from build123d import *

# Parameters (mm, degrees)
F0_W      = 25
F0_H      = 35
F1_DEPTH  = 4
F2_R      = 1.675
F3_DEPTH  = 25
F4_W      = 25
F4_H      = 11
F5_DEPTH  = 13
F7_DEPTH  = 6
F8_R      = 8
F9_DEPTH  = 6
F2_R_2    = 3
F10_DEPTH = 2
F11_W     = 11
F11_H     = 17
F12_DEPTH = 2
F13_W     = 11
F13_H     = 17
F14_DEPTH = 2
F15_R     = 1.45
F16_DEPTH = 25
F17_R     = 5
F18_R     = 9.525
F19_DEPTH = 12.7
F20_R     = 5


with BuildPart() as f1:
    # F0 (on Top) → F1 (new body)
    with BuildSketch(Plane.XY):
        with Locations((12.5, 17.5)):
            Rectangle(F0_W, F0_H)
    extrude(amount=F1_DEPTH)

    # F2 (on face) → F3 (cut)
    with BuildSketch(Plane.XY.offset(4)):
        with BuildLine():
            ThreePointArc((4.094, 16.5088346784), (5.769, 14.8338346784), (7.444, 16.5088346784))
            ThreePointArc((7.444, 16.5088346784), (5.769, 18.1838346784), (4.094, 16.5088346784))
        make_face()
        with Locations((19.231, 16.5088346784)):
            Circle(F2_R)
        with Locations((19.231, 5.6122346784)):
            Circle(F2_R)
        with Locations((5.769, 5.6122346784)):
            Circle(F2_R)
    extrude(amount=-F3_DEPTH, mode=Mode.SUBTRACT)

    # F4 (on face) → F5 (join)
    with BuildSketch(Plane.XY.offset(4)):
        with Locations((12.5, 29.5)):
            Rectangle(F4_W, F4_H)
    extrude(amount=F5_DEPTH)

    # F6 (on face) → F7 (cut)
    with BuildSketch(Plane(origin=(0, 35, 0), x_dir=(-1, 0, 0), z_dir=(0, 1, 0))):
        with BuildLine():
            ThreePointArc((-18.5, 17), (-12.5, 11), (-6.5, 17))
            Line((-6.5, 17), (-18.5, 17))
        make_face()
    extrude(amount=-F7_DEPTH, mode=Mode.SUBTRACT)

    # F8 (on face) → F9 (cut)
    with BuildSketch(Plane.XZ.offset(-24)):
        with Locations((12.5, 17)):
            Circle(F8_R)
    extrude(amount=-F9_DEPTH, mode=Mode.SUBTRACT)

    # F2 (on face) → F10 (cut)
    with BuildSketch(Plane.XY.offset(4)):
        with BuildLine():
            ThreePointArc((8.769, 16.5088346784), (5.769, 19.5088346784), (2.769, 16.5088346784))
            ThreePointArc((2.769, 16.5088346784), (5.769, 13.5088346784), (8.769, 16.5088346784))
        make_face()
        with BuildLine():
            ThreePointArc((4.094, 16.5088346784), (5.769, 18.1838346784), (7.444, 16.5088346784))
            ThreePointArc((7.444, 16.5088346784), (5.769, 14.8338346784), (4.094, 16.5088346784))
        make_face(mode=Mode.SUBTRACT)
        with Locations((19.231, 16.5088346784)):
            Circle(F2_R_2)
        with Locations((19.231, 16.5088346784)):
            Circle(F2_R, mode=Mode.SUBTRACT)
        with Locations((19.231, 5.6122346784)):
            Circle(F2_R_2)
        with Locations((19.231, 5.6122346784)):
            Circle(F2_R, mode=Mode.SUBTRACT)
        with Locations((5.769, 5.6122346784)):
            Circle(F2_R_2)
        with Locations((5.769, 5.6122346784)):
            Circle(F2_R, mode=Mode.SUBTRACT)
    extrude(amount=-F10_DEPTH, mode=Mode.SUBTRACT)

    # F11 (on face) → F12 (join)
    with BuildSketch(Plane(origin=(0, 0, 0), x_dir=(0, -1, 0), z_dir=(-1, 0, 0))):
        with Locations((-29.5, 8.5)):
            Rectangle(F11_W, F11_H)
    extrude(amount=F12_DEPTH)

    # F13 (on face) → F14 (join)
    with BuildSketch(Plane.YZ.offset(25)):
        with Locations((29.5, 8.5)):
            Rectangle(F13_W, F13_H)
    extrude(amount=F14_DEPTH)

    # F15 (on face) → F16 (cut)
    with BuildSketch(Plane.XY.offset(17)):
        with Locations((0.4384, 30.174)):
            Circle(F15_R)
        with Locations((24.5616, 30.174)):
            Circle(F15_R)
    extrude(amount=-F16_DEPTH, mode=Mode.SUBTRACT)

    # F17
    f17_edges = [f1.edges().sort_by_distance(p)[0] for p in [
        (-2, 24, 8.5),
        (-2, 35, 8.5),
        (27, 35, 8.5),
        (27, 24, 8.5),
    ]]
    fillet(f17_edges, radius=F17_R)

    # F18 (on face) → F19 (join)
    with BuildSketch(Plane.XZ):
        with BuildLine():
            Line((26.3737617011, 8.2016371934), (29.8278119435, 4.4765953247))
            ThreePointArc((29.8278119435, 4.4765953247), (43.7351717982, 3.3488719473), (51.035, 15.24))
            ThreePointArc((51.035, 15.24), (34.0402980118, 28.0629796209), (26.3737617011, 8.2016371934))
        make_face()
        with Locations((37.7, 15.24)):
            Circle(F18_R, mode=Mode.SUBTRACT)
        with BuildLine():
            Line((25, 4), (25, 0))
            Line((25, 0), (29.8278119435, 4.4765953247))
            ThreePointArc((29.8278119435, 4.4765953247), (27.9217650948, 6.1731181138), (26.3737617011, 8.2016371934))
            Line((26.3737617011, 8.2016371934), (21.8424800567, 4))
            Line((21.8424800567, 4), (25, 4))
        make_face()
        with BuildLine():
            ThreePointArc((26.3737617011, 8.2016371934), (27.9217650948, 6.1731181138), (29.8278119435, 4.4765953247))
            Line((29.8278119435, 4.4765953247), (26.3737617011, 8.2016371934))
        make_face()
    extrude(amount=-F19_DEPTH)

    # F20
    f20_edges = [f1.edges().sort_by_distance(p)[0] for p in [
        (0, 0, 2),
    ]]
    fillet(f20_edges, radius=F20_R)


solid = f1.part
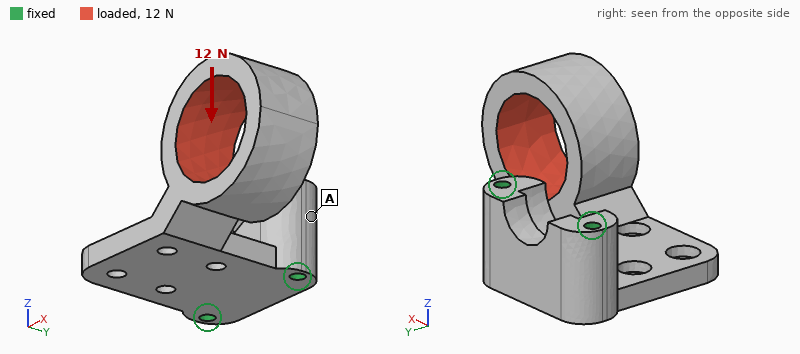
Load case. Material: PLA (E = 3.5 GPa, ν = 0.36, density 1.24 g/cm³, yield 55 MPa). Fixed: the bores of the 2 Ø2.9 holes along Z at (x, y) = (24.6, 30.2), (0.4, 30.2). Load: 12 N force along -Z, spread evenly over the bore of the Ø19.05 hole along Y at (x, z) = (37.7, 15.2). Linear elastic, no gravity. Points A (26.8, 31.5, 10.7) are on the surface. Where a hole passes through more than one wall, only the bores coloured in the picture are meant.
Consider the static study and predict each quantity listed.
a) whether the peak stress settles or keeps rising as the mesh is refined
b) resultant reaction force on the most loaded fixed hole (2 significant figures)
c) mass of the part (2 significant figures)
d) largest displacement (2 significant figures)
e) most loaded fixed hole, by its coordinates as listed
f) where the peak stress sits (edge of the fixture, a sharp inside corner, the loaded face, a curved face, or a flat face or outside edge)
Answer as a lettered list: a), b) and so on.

a) keeps rising
b) 21 N
c) 12 g
d) 0.67 mm
e) (24.6, 30.2)
f) a sharp inside corner
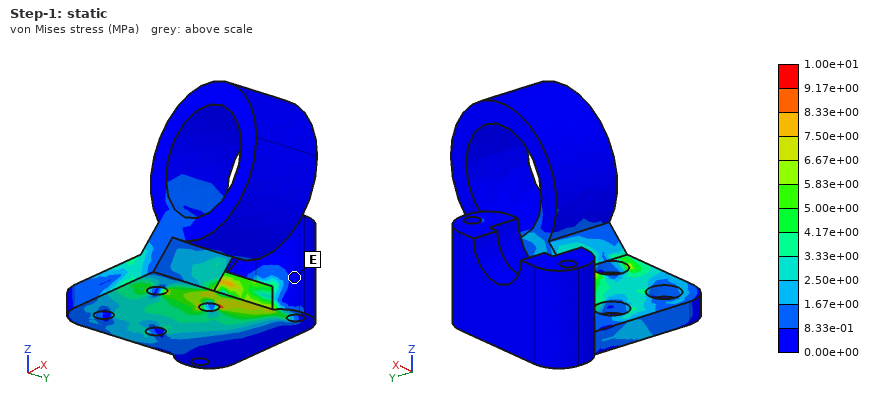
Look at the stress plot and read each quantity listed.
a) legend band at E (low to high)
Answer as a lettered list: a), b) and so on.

a) 0.00e+00 to 8.33e-01 MPa
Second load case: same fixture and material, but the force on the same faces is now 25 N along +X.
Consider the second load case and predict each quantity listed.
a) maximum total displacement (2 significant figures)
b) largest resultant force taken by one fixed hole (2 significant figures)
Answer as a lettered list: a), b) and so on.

a) 0.82 mm
b) 31 N
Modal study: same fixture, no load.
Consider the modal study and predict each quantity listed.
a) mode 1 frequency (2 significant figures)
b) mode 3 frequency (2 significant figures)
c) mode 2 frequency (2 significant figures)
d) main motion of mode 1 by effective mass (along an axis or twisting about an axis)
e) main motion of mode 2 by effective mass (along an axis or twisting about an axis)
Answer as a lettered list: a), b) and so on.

a) 340 Hz
b) 1500 Hz
c) 560 Hz
d) along Z
e) along Y
